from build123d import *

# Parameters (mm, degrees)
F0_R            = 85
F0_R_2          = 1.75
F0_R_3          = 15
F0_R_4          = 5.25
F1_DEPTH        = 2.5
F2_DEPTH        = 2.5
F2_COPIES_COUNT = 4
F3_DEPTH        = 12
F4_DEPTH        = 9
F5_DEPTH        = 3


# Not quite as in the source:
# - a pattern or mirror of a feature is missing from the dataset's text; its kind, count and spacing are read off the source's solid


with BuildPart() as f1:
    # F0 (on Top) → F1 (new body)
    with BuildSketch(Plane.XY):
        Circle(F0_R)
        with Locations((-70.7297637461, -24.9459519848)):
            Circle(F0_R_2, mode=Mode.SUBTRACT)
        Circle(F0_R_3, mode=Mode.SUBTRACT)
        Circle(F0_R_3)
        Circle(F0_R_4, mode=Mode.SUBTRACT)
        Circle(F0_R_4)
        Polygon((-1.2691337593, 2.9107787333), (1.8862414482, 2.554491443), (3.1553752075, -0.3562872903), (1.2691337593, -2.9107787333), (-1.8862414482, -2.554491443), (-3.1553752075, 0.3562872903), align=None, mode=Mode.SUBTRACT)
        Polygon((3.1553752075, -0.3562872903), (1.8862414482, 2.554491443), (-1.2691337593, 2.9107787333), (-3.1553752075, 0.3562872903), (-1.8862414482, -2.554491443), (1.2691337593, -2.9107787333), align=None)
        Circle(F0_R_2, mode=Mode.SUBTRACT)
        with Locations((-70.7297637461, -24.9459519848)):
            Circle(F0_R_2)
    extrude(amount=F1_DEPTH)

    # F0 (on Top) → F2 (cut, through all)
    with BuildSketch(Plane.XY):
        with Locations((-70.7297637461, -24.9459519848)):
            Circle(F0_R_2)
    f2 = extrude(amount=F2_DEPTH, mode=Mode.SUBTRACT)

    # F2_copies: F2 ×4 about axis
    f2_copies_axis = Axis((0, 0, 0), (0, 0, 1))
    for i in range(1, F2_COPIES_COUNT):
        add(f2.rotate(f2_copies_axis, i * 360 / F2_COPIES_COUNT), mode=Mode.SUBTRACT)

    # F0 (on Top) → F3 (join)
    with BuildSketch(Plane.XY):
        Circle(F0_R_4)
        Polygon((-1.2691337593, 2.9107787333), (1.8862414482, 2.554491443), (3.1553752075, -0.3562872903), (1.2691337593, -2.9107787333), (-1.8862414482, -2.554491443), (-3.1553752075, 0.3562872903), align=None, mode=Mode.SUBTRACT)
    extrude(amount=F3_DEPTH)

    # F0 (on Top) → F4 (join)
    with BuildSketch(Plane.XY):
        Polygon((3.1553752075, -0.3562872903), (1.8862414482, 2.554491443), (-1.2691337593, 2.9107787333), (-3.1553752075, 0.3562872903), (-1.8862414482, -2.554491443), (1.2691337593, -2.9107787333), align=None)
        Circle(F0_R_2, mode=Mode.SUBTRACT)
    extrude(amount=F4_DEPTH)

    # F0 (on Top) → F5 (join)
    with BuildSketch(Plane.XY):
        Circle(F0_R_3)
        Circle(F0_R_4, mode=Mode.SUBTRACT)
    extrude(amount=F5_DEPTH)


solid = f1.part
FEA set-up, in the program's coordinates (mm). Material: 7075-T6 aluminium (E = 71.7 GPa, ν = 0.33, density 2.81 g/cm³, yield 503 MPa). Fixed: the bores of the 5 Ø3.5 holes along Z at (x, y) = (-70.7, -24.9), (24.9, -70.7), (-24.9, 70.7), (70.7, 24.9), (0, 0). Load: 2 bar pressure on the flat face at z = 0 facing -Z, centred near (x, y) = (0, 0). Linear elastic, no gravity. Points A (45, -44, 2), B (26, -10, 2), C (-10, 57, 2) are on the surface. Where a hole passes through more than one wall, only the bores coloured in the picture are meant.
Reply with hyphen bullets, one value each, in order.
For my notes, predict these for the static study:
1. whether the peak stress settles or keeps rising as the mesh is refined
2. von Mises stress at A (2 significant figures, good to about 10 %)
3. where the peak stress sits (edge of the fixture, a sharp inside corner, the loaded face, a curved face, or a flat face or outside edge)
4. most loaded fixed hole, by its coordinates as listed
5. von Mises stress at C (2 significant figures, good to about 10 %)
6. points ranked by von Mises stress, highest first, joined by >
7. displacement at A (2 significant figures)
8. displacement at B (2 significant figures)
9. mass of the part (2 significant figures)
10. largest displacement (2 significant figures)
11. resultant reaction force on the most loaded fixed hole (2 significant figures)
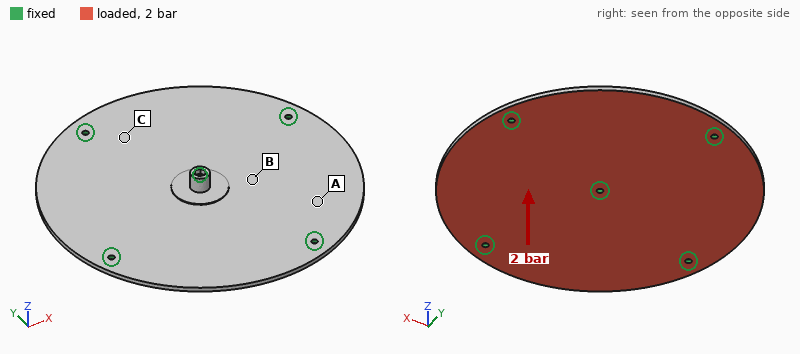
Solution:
- keeps rising
- 59 MPa
- edge of the fixture
- (0, 0)
- 93 MPa
- C > A > B
- 0.51 mm
- 0.22 mm
- 160 g
- 1.1 mm
- 1.3 kN
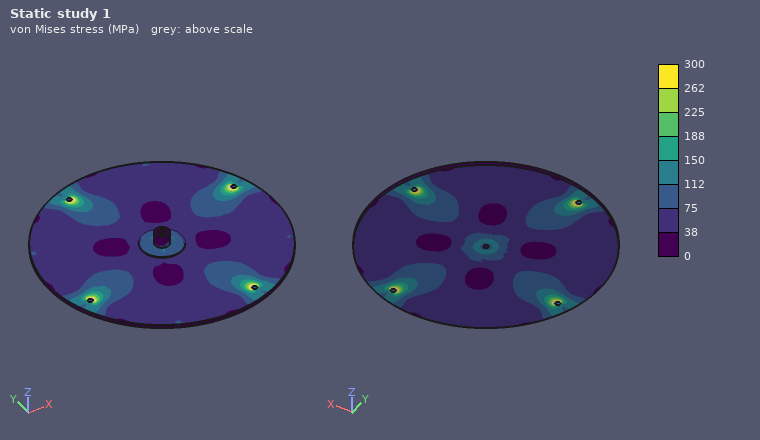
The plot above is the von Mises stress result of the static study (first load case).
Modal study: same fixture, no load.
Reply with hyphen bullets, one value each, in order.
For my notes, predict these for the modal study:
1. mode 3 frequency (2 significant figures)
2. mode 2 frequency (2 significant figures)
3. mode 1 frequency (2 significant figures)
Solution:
- 990 Hz
- 990 Hz
- 890 Hz
